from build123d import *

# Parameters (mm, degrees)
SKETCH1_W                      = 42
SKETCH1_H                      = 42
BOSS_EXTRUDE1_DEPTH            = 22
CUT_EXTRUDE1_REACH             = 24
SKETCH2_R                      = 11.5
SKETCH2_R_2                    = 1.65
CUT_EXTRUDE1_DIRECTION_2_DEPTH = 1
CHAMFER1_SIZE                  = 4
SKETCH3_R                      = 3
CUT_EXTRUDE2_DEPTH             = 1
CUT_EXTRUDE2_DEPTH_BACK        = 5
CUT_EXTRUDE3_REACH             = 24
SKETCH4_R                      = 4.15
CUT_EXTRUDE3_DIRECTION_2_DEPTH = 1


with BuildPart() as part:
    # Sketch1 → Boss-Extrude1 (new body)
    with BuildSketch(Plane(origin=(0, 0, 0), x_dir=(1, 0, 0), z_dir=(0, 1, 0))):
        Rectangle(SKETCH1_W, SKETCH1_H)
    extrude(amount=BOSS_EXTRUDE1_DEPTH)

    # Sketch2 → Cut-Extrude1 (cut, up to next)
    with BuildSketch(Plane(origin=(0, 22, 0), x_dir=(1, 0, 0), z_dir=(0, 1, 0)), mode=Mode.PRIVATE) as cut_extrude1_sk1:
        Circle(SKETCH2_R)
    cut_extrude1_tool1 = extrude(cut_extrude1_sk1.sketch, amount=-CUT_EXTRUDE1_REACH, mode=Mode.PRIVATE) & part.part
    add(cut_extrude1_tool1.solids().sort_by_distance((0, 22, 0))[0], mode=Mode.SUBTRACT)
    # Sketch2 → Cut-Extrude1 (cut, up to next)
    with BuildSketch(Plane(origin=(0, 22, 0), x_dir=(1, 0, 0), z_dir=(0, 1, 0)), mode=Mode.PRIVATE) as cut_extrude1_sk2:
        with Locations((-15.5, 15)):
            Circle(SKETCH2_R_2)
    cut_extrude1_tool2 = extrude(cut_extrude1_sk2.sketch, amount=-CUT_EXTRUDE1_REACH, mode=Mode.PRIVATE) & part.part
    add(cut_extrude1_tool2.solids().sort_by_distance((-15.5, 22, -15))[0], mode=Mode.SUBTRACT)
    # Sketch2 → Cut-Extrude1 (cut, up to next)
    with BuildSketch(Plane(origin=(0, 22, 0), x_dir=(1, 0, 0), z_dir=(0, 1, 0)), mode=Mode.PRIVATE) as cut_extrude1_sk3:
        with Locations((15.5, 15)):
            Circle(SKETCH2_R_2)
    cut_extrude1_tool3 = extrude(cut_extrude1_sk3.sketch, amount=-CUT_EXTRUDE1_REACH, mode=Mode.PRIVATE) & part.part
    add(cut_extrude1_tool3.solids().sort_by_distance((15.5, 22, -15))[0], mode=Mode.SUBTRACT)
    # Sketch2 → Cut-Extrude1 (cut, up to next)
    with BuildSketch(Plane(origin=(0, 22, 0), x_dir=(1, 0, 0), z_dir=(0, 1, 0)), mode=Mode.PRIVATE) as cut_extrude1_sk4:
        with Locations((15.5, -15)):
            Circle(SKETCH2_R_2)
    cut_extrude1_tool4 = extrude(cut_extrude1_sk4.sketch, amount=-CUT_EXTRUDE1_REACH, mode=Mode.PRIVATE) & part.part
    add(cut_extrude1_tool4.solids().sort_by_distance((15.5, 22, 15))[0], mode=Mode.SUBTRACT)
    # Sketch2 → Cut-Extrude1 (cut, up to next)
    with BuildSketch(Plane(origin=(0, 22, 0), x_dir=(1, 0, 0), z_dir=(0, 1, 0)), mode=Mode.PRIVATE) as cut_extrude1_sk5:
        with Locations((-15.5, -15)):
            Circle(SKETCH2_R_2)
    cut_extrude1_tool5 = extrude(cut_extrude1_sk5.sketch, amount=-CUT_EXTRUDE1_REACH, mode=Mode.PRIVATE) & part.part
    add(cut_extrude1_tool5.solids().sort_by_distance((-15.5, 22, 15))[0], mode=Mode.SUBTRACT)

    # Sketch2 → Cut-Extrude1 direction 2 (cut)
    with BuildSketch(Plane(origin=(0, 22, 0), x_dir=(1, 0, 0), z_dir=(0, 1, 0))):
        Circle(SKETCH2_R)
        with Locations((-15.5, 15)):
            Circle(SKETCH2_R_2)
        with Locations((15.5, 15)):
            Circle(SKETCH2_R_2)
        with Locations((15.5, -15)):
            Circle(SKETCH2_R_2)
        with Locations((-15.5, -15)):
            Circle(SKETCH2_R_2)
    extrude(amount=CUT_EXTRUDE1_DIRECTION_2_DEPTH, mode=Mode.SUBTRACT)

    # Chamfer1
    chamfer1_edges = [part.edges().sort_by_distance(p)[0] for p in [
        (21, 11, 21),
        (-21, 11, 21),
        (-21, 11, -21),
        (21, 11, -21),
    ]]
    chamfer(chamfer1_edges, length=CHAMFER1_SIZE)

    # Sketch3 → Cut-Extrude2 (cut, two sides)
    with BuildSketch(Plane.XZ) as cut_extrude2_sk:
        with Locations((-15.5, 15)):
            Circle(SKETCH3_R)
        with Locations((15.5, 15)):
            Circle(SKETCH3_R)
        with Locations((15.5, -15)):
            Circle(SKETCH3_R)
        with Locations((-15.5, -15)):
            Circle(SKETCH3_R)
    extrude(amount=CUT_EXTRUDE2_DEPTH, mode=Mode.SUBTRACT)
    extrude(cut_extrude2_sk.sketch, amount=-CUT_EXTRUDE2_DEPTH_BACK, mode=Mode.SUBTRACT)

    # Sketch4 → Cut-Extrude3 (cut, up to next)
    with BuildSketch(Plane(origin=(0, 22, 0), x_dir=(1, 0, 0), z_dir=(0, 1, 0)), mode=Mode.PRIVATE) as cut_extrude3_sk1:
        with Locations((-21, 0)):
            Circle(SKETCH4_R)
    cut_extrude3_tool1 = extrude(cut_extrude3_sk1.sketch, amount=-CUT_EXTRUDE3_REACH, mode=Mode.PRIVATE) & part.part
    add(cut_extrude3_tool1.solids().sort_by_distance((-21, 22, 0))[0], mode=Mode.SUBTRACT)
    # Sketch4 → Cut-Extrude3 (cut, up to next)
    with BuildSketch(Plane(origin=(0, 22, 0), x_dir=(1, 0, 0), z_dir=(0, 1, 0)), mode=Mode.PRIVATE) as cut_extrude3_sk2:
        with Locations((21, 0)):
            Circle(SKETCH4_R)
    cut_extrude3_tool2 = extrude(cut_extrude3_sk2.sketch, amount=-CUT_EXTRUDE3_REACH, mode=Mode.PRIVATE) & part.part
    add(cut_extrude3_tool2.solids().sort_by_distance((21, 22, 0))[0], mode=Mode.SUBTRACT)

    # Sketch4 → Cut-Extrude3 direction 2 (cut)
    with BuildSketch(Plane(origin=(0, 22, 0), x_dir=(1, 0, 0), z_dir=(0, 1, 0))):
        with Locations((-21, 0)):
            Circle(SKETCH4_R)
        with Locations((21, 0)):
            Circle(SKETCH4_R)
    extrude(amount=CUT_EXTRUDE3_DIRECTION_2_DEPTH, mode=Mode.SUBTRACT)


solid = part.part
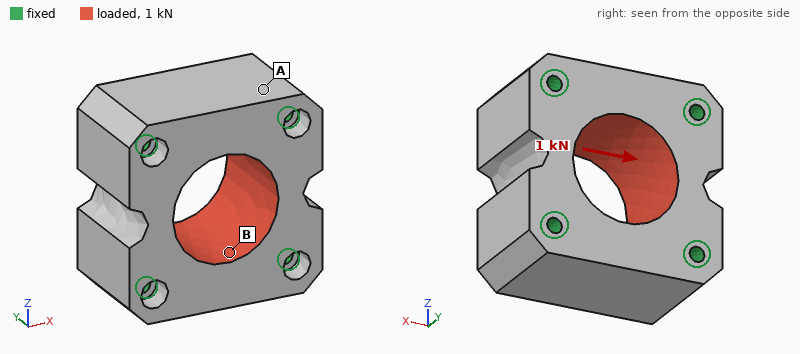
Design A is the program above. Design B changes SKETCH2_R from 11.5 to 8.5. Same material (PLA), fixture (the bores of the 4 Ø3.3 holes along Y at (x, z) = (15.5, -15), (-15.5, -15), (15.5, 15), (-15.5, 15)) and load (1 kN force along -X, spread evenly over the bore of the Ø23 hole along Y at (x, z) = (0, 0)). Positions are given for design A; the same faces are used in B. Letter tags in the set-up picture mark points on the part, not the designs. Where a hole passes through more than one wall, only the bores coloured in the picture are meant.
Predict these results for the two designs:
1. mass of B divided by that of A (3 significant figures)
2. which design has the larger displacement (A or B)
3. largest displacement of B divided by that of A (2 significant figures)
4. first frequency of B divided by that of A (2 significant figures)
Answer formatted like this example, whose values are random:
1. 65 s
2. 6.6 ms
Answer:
1. 1.16
2. A
3. 0.80
4. 1.3
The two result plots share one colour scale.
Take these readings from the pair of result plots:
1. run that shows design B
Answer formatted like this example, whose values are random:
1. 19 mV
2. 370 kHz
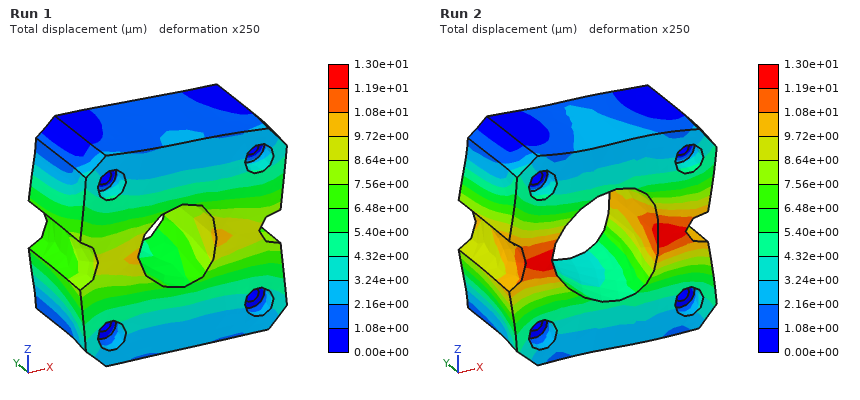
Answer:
1. Run 1
